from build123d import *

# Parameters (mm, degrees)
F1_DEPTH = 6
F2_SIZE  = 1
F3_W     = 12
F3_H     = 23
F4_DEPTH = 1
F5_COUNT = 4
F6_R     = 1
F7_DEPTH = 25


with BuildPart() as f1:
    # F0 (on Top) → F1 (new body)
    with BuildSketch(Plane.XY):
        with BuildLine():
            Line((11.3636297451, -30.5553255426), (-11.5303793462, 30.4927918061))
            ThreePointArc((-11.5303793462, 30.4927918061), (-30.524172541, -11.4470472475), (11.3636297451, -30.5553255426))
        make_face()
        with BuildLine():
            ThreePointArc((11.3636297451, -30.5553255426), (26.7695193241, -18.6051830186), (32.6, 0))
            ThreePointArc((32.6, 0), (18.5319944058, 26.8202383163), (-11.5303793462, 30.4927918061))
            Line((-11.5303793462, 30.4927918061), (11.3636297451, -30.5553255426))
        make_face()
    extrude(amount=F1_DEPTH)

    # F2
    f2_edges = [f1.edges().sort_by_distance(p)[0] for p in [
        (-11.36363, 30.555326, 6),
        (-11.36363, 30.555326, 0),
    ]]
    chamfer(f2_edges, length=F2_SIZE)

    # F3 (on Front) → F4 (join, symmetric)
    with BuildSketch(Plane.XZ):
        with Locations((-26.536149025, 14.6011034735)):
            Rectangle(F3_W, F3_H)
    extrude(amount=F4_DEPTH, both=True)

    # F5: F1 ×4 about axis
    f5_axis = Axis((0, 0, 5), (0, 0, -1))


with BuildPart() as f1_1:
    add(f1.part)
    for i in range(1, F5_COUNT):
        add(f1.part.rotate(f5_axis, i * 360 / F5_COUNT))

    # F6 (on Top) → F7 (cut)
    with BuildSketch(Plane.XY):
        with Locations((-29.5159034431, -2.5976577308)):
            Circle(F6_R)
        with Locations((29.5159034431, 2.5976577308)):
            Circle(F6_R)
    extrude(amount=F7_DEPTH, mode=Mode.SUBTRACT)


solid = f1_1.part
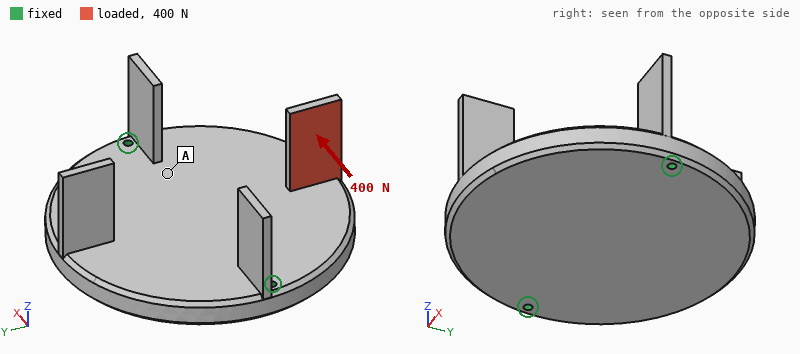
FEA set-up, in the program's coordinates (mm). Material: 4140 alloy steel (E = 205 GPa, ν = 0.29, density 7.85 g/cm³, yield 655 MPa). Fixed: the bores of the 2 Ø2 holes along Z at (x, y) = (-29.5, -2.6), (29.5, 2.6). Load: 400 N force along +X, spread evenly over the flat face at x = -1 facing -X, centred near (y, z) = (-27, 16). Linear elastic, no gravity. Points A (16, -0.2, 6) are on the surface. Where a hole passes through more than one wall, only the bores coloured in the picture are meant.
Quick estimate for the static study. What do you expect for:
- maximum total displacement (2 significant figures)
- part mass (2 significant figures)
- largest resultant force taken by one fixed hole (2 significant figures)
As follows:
0.28 mm
170 g
300 N
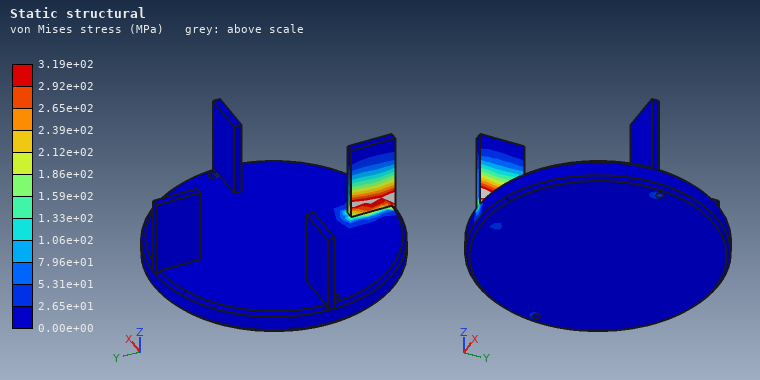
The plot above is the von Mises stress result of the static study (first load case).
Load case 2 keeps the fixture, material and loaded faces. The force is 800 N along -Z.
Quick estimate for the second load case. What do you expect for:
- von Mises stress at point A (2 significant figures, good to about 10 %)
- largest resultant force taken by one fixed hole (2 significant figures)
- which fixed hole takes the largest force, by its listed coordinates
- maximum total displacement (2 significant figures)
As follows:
40 MPa
450 N
(-29.5, -2.6)
0.13 mm
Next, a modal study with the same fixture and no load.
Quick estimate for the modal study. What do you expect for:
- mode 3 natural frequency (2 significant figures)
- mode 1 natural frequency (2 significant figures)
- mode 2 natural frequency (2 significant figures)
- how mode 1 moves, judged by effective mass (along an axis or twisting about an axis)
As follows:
3800 Hz
2500 Hz
3700 Hz
twisting about X
